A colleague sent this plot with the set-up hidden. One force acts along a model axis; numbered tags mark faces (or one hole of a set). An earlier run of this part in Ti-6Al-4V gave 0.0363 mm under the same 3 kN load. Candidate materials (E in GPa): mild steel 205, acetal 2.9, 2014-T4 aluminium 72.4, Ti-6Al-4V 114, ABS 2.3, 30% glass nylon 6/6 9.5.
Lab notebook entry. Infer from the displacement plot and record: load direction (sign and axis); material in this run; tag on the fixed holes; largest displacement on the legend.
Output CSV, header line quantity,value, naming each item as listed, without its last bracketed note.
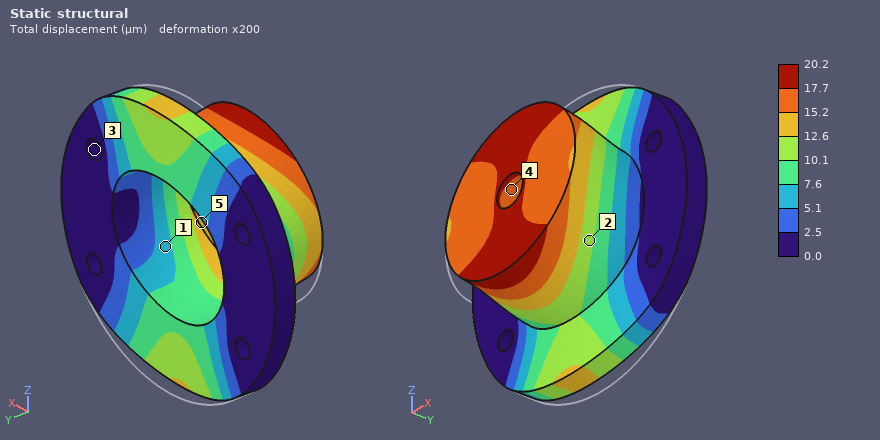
quantity,value
load direction,+Z
material in this run,mild steel
tag on the fixed holes,3
largest displacement on the legend,20.2 µm
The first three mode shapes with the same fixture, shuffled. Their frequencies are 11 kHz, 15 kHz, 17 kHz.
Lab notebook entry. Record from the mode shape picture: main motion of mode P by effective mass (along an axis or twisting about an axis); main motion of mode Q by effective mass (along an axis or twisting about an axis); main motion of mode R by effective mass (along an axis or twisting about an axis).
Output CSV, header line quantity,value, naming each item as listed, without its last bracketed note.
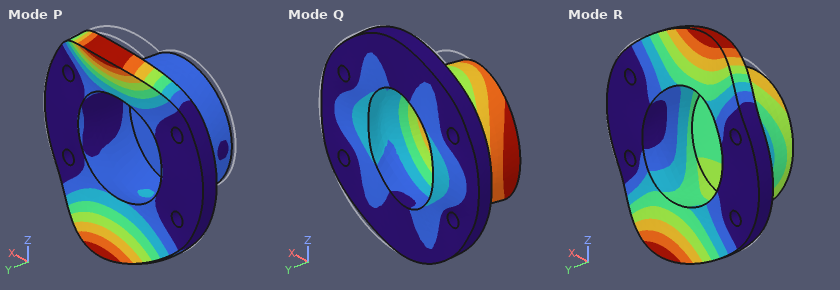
quantity,value
main motion of mode P by effective mass,along Y
main motion of mode Q by effective mass,along X
main motion of mode R by effective mass,along Z
